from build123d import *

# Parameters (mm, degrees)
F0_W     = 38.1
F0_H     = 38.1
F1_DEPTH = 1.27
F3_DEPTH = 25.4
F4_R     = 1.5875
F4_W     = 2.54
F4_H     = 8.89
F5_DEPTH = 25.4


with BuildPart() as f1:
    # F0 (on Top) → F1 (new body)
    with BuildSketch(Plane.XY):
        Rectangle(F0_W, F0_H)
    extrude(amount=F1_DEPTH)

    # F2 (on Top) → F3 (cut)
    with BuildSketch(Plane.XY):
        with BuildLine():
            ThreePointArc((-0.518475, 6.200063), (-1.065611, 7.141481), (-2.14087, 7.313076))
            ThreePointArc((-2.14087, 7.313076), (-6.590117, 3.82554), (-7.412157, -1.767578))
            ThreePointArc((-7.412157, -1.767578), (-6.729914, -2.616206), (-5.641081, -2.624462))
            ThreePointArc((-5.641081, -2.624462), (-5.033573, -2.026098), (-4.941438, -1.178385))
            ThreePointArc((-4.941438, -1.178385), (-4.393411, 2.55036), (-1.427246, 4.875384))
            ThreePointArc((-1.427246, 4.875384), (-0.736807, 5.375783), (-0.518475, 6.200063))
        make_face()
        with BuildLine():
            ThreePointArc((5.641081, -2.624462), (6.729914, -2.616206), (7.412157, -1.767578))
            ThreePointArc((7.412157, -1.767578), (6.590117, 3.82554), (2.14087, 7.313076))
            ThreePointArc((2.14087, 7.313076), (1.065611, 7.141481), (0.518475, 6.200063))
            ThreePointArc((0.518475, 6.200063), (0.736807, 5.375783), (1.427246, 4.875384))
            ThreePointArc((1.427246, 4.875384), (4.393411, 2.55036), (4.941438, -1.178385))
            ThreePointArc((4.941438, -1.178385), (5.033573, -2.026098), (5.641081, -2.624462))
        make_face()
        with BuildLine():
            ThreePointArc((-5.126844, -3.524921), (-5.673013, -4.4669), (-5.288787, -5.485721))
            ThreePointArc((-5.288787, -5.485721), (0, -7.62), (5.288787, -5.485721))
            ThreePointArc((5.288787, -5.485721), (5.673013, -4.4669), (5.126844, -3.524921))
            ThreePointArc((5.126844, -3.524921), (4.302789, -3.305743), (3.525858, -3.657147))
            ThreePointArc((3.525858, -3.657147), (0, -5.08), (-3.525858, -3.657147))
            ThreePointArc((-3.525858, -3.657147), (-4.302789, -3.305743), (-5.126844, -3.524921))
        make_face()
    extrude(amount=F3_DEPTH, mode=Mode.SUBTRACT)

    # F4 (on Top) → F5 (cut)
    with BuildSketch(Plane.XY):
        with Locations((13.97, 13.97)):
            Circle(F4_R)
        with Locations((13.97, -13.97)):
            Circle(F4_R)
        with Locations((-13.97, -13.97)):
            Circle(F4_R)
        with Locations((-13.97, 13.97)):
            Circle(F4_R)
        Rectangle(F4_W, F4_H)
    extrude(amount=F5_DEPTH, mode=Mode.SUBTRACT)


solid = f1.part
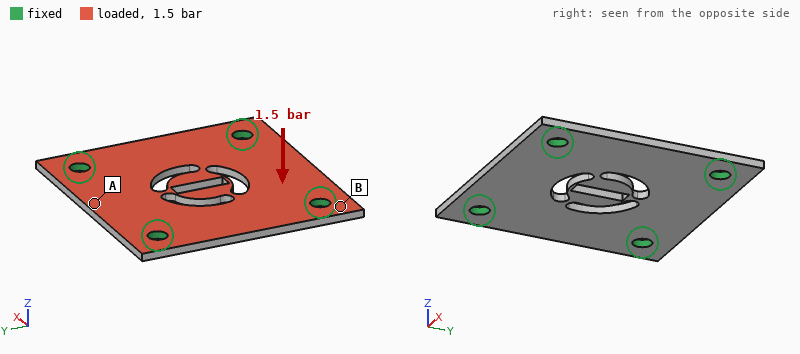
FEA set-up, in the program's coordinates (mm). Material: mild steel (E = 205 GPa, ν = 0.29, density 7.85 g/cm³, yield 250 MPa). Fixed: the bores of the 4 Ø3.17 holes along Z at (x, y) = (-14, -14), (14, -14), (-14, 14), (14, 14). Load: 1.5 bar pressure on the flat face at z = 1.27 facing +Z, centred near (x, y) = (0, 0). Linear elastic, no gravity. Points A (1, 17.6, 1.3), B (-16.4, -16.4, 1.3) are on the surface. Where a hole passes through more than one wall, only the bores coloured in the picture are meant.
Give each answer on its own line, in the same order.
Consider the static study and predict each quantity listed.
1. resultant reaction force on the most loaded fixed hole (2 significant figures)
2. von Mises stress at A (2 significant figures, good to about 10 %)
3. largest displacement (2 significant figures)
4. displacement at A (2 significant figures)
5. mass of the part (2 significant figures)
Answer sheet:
49 N
17 MPa
15 µm
5.1 µm
13 g
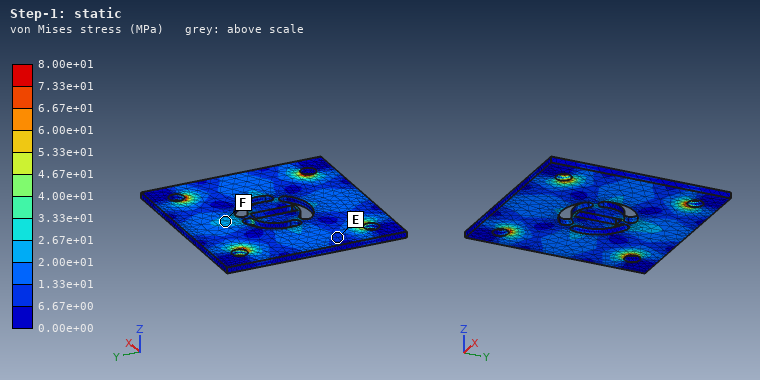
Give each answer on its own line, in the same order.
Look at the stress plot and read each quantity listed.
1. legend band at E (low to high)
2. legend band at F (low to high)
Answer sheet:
6.67e+00 to 1.33e+01 MPa
2.00e+01 to 2.67e+01 MPa
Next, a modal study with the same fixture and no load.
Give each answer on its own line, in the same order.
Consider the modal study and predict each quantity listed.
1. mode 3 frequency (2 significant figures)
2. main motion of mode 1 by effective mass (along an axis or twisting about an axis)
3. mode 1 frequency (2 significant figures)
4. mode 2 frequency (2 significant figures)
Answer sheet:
10000 Hz
along Z
6700 Hz
9900 Hz
